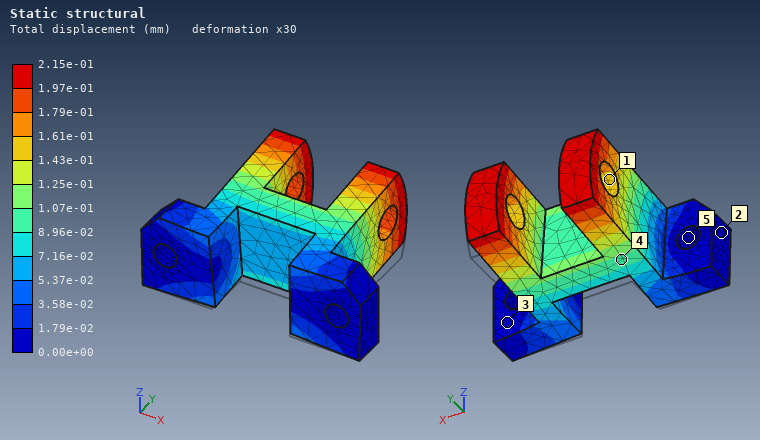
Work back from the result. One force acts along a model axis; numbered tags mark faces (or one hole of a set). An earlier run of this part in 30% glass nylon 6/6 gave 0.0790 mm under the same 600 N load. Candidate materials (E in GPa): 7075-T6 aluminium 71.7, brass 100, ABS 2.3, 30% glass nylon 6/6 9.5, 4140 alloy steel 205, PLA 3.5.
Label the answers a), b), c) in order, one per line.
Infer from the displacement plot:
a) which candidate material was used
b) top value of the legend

a) PLA
b) 2.15e-01 mm
